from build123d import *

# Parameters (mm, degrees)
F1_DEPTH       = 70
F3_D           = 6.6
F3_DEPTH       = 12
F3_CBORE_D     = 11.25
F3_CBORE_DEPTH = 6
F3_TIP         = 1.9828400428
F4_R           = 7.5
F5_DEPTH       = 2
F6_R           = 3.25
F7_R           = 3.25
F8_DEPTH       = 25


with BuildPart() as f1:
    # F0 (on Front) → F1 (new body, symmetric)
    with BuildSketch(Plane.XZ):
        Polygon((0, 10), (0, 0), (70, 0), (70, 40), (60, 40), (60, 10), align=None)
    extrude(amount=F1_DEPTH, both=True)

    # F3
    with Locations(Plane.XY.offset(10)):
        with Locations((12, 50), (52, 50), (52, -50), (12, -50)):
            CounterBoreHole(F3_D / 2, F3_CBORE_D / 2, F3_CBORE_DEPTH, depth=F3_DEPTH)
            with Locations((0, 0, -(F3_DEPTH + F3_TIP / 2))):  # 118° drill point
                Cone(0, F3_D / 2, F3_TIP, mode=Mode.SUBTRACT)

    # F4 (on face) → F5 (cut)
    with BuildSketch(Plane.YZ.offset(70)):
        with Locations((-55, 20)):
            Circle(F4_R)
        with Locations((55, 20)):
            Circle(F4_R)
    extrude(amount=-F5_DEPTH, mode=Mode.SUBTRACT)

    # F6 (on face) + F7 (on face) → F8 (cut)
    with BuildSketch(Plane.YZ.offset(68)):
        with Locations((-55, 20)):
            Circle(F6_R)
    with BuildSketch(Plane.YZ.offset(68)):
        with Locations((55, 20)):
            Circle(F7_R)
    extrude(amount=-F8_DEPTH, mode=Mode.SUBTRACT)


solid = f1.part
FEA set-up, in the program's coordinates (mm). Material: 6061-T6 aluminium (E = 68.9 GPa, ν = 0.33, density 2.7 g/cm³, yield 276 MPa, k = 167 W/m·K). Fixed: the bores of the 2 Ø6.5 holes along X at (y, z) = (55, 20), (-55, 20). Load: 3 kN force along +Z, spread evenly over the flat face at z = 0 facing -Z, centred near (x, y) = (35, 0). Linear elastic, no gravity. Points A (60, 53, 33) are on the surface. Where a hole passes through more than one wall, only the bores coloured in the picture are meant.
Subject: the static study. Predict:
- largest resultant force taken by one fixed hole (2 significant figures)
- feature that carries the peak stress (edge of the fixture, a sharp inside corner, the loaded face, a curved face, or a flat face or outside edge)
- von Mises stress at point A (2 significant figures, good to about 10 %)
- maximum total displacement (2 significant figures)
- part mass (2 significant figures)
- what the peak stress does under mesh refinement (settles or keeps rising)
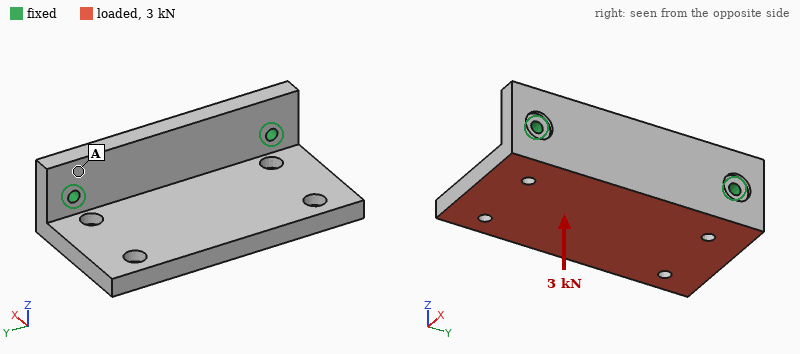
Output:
1.5 kN
edge of the fixture
23 MPa
0.37 mm
370 g
keeps rising
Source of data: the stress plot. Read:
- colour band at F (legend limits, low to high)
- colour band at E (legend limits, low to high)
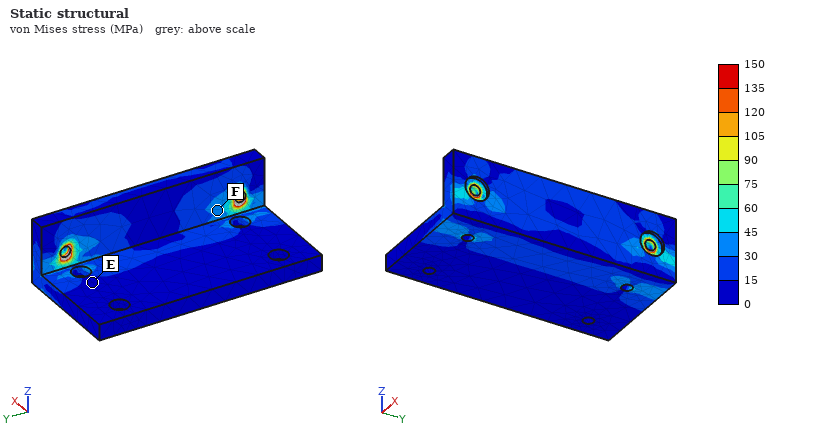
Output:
30 to 45 MPa
0 to 15 MPa
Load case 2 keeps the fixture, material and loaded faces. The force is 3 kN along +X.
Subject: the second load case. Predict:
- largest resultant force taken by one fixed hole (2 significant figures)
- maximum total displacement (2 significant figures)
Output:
1.5 kN
0.15 mm
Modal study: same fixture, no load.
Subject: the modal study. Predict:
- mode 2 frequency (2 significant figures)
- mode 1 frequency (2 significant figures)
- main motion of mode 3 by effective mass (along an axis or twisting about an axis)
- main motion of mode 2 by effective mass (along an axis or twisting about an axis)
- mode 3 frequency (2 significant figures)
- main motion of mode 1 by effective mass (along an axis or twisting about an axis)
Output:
2200 Hz
1100 Hz
along X
twisting about X
4100 Hz
along Z
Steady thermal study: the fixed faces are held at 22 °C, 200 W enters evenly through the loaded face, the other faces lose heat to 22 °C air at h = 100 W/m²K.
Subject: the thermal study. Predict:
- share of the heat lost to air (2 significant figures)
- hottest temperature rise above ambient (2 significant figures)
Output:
31 %
42 K
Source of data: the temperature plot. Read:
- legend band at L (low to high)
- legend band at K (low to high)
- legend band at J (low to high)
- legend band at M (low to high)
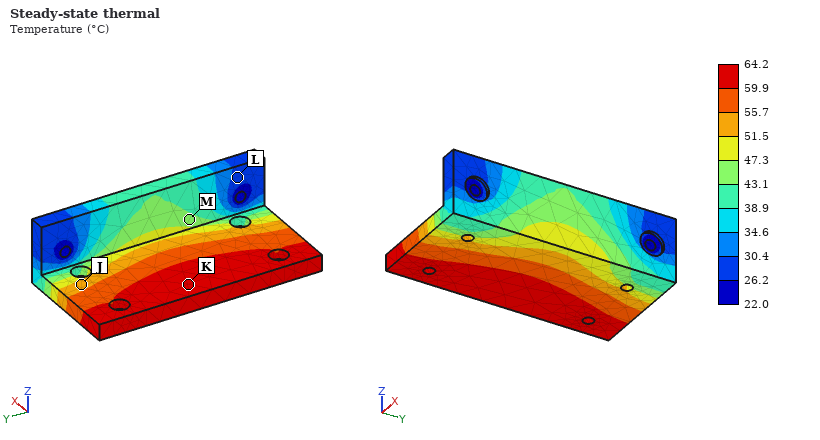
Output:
26.2 to 30.4 °C
59.9 to 64.2 °C
51.5 to 55.7 °C
43.1 to 47.3 °C
